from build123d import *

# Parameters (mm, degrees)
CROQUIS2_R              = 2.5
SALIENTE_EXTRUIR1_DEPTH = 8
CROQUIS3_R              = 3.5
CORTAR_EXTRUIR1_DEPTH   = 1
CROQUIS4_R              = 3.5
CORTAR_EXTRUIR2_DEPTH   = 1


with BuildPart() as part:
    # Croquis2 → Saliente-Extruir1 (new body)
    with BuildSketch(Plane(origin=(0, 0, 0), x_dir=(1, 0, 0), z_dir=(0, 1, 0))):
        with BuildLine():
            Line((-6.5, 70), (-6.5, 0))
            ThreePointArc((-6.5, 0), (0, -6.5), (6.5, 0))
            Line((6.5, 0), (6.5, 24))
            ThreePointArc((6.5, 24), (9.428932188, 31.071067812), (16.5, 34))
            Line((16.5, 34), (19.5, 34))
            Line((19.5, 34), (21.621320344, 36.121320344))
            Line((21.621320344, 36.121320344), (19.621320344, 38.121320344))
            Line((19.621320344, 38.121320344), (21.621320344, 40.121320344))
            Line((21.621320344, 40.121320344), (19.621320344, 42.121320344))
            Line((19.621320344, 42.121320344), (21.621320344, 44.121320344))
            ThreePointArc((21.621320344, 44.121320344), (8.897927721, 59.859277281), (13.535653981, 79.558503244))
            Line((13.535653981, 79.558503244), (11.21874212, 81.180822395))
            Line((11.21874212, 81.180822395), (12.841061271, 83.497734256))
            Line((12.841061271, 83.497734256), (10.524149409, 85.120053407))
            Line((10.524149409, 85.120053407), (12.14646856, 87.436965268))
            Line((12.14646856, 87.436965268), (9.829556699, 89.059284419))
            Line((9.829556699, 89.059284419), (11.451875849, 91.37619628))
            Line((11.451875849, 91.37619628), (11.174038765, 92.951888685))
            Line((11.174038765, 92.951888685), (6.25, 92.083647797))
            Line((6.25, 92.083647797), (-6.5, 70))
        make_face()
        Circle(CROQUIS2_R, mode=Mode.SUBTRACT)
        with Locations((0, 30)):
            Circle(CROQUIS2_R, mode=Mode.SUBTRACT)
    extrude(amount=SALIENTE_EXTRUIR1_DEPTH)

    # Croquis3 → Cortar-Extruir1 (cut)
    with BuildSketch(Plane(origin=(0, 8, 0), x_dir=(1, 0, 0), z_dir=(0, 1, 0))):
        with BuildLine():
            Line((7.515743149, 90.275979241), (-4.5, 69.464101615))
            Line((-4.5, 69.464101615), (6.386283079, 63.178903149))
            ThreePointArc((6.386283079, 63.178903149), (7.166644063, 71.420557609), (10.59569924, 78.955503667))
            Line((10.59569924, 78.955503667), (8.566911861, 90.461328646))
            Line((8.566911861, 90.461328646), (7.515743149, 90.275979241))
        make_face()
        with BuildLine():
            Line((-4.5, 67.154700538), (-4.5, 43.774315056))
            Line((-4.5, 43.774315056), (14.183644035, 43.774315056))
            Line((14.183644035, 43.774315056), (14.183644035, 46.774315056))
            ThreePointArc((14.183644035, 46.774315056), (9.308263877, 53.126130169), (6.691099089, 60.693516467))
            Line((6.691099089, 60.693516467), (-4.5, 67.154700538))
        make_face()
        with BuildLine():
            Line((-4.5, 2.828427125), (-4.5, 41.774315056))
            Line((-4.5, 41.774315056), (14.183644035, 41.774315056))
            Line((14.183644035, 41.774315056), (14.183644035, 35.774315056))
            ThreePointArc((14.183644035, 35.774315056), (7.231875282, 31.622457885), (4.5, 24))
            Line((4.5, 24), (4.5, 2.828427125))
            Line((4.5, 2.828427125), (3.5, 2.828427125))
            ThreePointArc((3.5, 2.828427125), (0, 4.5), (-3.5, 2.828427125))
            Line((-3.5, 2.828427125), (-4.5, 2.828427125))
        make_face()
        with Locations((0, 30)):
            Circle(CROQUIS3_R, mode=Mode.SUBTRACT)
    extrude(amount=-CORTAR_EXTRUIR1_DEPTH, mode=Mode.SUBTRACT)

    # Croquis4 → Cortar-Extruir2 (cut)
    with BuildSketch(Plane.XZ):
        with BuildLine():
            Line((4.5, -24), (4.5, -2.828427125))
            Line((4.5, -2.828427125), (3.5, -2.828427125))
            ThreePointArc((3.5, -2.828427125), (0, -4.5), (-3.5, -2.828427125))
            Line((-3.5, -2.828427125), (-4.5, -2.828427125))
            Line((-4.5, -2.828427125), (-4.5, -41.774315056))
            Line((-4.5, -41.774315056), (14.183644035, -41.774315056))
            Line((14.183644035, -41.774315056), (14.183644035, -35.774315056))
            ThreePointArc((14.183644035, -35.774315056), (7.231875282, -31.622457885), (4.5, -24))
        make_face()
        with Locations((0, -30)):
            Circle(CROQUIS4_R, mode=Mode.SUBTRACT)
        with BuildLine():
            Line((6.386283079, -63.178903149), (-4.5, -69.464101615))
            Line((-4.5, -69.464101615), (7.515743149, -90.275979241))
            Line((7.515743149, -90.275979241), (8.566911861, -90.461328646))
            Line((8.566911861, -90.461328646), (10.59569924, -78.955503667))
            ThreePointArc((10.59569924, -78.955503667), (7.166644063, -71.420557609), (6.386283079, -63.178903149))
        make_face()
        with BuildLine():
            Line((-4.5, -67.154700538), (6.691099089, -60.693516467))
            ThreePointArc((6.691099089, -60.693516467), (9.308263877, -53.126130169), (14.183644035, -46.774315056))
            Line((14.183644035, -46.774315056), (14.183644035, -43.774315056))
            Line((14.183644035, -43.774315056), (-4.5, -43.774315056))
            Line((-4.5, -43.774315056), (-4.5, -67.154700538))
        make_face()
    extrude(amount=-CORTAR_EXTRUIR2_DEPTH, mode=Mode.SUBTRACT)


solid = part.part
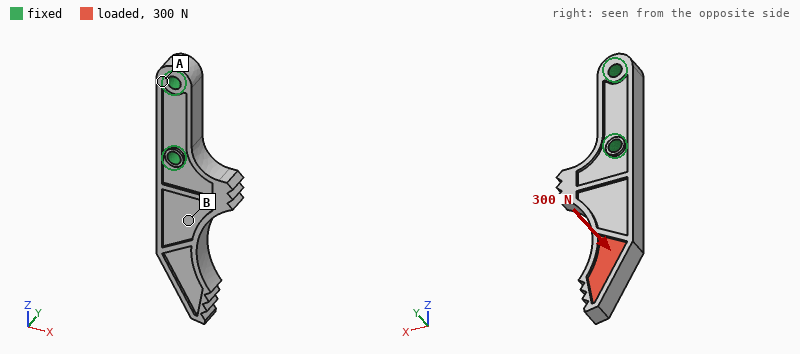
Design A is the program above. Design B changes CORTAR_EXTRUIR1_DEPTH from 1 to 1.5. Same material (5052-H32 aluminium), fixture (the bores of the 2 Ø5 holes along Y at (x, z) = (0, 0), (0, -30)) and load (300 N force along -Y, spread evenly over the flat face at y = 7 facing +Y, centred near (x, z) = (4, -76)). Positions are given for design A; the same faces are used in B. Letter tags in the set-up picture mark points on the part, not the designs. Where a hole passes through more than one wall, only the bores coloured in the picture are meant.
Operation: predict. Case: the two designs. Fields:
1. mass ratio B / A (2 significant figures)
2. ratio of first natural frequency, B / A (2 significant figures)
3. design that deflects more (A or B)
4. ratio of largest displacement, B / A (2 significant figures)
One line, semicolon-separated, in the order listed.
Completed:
0.96; 0.94; B; 1.2
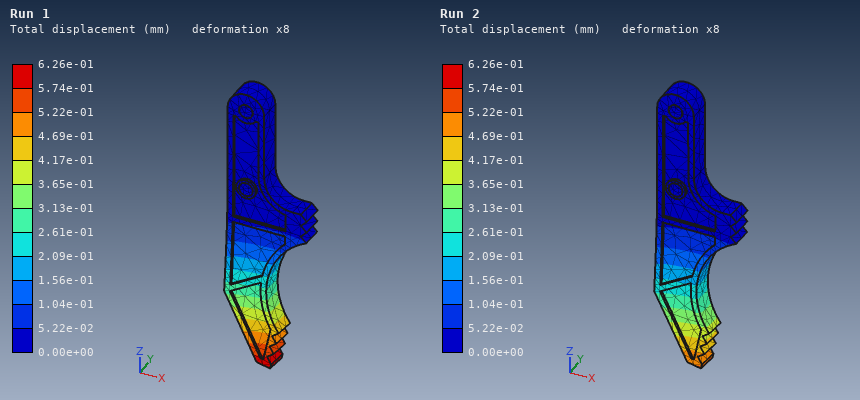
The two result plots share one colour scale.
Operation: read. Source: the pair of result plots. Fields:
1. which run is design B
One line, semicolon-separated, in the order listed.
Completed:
Run 1
